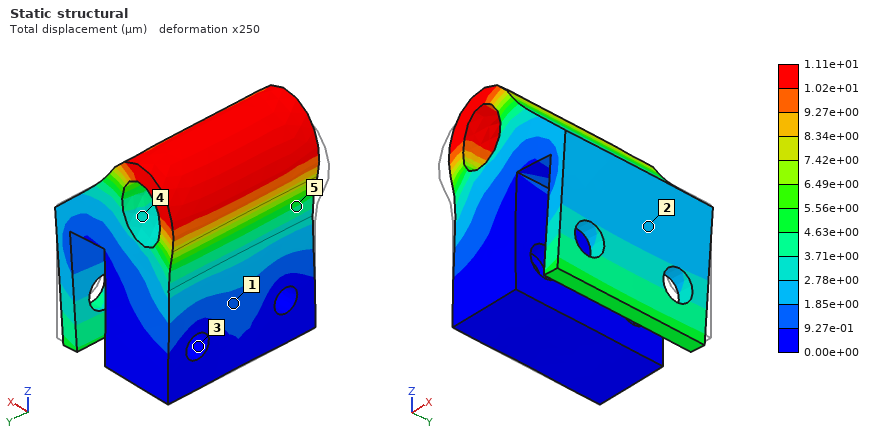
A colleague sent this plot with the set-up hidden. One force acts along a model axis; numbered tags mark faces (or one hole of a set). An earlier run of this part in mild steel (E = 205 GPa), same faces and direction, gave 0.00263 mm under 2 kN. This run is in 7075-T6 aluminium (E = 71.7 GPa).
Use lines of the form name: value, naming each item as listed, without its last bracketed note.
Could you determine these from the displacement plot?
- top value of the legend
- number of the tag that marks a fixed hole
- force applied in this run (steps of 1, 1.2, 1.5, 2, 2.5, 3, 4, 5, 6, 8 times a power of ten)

top value of the legend: 1.11e+01 µm
number of the tag that marks a fixed hole: 3
force applied in this run: 3 kN
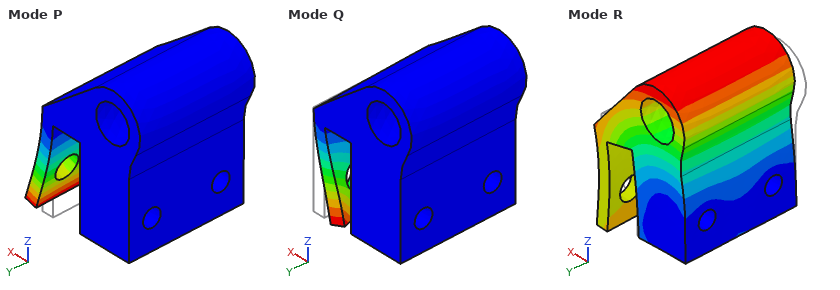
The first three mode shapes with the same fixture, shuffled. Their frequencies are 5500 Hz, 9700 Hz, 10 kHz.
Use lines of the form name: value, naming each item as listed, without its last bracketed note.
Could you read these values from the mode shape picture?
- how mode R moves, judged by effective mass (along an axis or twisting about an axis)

how mode R moves, judged by effective mass: along X
